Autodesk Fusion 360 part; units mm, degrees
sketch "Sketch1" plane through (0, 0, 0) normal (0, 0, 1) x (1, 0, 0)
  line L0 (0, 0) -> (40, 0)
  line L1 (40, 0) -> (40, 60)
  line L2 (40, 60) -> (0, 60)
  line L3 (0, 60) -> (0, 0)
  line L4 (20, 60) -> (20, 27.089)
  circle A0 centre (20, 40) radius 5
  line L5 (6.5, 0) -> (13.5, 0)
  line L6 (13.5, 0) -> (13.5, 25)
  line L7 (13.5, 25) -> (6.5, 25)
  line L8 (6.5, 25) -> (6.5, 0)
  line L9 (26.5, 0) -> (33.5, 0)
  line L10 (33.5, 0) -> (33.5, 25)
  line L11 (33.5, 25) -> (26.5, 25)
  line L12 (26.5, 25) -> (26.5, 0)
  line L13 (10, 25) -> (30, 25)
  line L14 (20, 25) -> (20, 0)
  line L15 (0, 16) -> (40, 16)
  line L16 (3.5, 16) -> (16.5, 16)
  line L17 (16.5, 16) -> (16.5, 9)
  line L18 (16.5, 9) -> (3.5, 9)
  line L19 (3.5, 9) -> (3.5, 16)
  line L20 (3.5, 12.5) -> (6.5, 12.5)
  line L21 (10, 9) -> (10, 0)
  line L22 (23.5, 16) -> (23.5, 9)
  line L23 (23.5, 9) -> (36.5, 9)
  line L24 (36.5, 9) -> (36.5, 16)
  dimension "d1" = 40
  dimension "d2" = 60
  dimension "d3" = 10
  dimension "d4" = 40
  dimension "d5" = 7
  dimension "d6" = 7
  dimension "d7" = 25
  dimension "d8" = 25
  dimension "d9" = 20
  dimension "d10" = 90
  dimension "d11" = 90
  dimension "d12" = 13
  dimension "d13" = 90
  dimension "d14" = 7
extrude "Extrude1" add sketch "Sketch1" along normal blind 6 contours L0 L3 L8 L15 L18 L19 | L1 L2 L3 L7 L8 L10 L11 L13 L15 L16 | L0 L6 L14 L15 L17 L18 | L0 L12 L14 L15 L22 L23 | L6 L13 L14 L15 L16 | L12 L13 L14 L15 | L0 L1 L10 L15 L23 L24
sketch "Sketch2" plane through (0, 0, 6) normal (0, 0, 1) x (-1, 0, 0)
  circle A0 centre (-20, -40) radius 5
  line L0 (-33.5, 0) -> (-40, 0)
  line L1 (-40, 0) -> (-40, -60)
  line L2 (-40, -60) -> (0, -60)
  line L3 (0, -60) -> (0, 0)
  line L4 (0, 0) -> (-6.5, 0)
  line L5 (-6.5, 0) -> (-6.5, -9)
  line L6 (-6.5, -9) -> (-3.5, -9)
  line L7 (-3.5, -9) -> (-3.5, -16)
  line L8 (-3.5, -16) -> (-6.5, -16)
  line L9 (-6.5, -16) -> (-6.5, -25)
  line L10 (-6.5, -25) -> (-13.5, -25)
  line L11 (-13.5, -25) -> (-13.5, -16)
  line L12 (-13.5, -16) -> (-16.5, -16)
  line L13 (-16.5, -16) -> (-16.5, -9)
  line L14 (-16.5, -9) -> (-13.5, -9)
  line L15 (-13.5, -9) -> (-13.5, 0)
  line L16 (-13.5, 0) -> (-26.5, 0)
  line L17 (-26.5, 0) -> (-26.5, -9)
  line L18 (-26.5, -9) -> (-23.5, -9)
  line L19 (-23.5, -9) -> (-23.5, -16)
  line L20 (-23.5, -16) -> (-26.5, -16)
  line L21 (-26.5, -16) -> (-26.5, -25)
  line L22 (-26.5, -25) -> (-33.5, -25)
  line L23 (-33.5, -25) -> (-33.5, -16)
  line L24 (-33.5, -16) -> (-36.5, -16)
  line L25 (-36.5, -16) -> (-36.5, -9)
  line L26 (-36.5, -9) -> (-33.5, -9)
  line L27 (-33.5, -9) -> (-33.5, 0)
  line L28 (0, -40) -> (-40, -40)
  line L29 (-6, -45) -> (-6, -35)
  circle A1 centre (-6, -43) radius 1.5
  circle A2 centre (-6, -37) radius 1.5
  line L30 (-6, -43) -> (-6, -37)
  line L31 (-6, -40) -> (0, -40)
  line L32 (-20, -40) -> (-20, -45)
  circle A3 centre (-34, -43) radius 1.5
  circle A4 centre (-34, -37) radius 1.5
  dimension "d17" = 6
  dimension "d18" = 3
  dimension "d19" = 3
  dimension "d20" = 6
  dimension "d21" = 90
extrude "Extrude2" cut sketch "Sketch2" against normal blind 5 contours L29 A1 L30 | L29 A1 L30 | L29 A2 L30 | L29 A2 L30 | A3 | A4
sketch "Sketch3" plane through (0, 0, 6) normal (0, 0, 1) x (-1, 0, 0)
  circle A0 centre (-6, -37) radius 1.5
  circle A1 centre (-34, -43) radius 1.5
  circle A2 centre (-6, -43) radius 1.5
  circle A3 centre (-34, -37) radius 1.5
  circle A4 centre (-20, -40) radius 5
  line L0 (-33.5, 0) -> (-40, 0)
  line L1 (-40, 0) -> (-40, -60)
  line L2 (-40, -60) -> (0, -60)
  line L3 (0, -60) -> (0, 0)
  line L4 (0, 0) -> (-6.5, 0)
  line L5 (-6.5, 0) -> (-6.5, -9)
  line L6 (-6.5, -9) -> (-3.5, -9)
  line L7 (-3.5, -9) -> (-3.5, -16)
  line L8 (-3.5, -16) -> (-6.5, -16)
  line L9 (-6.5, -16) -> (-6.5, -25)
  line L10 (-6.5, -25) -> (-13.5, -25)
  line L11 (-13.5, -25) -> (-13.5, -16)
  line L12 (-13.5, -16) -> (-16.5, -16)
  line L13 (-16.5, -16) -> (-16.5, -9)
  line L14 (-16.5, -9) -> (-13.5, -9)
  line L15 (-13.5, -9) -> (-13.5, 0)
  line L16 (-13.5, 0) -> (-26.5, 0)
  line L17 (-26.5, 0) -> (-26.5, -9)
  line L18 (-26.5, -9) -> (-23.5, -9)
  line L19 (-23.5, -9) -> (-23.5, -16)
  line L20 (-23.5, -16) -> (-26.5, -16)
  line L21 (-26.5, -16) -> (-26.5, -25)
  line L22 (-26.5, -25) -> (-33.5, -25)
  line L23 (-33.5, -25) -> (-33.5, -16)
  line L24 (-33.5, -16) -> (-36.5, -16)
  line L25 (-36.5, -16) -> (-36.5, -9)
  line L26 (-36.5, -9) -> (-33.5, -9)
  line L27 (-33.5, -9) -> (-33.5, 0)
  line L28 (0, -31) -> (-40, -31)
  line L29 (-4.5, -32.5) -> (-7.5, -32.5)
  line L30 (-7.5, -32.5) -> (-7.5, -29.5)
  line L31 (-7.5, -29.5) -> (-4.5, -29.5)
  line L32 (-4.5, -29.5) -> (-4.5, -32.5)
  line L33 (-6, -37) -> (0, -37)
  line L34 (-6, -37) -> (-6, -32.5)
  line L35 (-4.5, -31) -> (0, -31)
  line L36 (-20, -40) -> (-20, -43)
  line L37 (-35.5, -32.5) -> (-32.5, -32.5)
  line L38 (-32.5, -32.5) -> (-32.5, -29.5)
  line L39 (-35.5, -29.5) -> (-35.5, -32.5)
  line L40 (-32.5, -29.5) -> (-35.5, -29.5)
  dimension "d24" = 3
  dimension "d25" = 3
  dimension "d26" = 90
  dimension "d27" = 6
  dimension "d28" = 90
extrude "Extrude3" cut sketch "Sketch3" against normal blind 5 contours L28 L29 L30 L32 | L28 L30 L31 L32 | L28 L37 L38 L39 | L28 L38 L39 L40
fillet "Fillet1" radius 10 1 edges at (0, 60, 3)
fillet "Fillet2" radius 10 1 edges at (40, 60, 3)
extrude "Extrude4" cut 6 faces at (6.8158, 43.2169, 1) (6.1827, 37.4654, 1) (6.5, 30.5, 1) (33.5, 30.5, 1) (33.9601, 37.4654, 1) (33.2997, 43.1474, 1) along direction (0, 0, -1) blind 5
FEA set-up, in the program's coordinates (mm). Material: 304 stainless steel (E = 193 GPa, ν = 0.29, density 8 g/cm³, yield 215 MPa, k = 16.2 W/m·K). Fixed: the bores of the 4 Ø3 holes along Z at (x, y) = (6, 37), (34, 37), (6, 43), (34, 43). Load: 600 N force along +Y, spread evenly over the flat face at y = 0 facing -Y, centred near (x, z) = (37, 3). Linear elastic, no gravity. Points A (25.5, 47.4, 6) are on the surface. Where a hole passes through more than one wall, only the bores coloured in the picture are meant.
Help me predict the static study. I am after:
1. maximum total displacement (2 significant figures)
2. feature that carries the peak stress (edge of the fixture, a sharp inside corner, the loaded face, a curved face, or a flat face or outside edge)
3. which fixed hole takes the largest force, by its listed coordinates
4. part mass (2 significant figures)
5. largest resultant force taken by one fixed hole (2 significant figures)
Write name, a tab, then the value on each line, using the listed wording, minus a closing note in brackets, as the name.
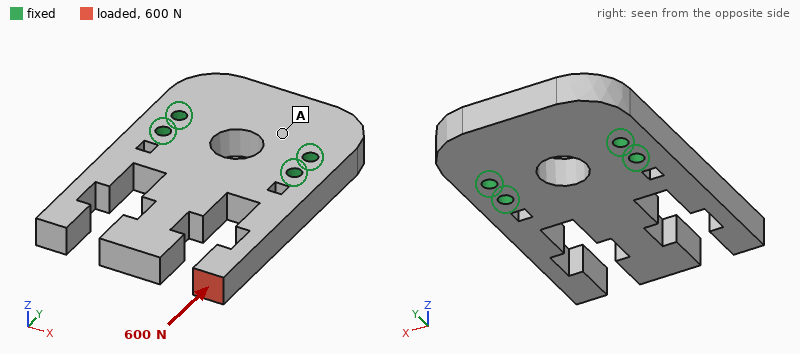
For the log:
maximum total displacement	26 µm
feature that carries the peak stress	a sharp inside corner
which fixed hole takes the largest force, by its listed coordinates	(34, 37)
part mass	86 g
largest resultant force taken by one fixed hole	470 N
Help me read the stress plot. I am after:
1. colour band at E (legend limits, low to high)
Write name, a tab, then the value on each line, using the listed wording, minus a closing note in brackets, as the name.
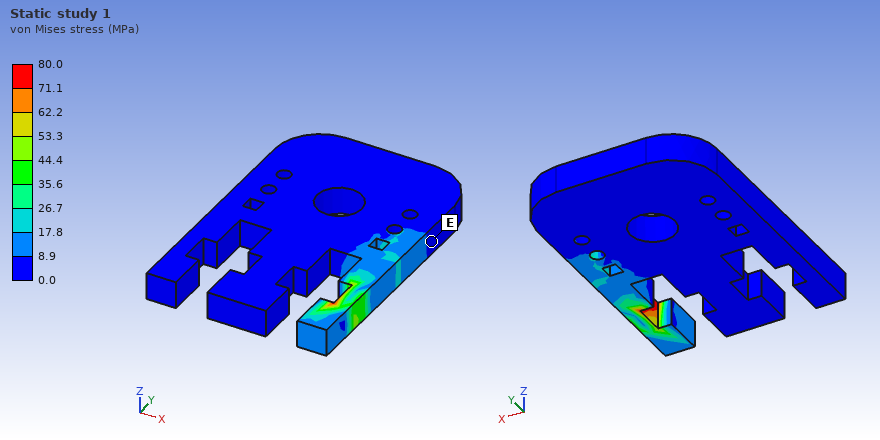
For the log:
colour band at E	0.0 to 8.9 MPa
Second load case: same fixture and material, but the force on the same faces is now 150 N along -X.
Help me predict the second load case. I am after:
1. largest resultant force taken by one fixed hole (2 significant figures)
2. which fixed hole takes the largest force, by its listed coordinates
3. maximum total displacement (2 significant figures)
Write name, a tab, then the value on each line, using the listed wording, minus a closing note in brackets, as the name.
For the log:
largest resultant force taken by one fixed hole	180 N
which fixed hole takes the largest force, by its listed coordinates	(6, 37)
maximum total displacement	99 µm
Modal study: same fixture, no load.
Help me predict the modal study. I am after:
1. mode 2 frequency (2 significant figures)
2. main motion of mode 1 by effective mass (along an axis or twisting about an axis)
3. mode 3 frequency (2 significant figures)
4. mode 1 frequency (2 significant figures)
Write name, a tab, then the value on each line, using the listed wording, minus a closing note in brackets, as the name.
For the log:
mode 2 frequency	4200 Hz
main motion of mode 1 by effective mass	along Z
mode 3 frequency	4600 Hz
mode 1 frequency	3500 Hz
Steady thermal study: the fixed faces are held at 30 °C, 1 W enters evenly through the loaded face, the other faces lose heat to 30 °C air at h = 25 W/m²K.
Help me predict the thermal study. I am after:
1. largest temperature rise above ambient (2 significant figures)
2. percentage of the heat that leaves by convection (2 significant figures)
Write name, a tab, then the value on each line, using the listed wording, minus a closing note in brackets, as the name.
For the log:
largest temperature rise above ambient	46 K
percentage of the heat that leaves by convection	47 %
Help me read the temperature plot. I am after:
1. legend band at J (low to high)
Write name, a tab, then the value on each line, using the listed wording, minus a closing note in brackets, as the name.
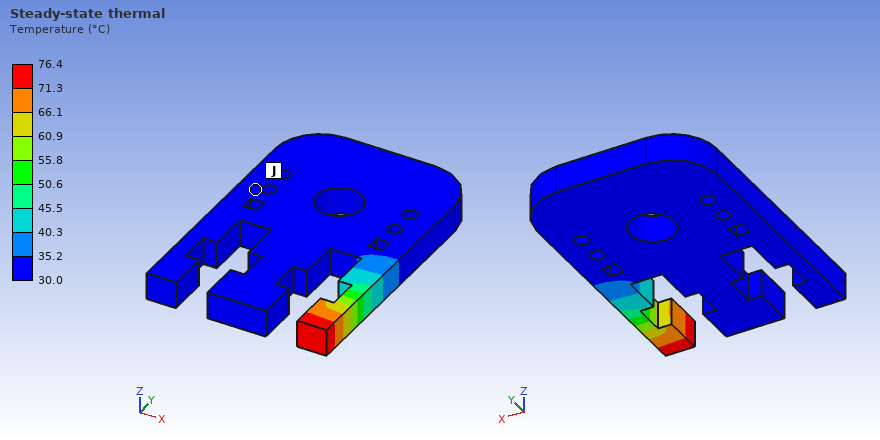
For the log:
legend band at J	30.0 to 35.2 °C
